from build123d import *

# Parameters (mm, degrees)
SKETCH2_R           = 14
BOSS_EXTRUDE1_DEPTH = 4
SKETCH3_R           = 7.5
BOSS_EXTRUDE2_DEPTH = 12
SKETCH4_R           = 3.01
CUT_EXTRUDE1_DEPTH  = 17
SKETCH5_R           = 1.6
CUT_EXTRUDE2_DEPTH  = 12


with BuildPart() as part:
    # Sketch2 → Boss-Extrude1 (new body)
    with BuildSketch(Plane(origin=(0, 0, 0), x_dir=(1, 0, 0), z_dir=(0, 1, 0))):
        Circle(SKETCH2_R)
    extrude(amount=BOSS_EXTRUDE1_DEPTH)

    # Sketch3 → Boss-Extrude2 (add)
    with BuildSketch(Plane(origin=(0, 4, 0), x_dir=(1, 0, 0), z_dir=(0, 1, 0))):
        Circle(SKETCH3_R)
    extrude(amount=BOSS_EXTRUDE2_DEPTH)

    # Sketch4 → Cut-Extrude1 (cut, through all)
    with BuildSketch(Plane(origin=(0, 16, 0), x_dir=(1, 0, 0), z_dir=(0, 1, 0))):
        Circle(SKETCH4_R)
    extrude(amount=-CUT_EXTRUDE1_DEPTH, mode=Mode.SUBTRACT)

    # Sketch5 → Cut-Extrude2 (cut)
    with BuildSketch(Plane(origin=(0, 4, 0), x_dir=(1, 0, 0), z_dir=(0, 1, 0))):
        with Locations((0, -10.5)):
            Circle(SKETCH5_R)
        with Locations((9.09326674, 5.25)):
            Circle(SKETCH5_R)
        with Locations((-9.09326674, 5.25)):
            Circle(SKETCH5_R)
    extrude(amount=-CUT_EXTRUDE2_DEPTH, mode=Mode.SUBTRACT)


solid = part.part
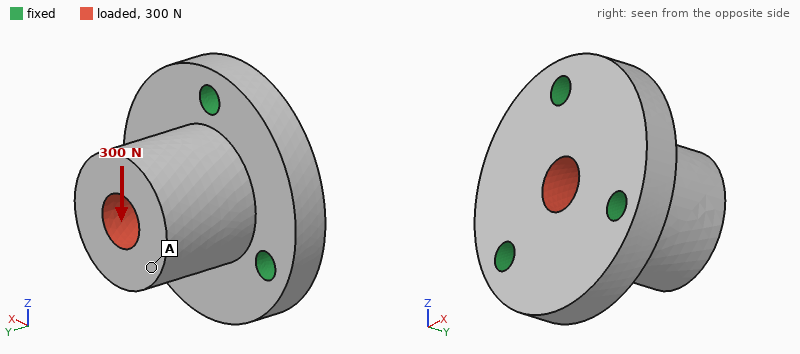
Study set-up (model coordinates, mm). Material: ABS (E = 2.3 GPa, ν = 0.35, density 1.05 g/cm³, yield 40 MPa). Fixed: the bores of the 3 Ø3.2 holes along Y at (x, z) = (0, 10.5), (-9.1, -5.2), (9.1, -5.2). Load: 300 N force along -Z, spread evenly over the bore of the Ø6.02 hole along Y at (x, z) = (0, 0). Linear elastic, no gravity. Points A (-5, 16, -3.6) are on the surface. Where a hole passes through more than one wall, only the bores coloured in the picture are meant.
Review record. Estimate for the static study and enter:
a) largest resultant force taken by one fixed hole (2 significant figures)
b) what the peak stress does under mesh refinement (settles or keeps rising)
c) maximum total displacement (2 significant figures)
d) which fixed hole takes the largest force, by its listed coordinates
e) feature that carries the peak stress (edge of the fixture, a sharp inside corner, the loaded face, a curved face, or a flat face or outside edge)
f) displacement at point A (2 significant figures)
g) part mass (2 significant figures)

170 N
keeps rising
72 µm
(0, 10.5)
edge of the fixture
65 µm
4.2 g
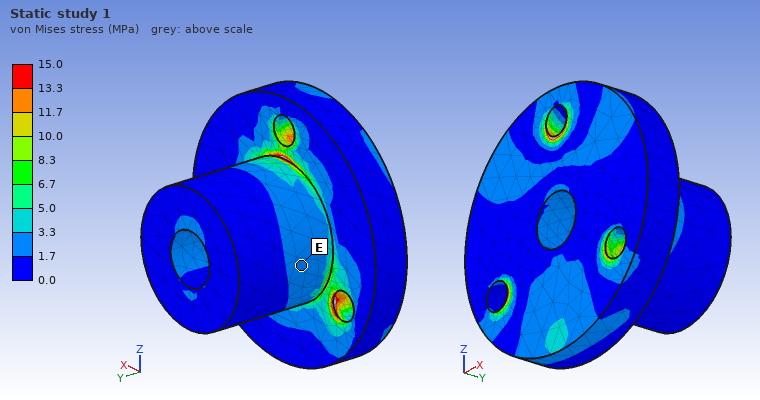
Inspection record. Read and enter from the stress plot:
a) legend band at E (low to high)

1.7 to 3.3 MPa
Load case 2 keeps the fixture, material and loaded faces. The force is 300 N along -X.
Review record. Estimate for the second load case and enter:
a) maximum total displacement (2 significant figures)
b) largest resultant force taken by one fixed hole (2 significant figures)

71 µm
150 N
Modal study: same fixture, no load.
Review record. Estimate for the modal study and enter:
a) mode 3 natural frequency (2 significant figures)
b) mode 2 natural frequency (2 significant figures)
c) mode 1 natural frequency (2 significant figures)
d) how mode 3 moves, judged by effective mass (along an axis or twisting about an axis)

10 kHz
7300 Hz
7300 Hz
along Y
